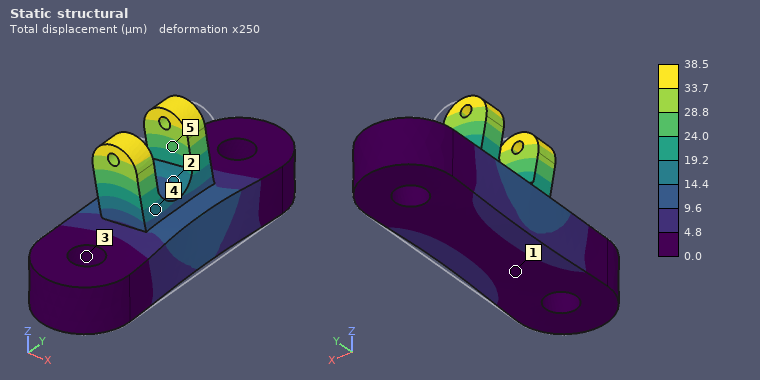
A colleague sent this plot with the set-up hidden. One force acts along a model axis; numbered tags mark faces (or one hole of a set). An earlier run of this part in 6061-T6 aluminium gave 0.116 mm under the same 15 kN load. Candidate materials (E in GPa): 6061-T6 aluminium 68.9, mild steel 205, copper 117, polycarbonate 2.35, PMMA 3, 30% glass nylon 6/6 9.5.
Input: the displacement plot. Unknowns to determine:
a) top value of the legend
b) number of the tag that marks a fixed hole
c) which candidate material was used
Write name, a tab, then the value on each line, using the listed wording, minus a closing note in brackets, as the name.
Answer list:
top value of the legend	38.5 µm
number of the tag that marks a fixed hole	3
which candidate material was used	mild steel
